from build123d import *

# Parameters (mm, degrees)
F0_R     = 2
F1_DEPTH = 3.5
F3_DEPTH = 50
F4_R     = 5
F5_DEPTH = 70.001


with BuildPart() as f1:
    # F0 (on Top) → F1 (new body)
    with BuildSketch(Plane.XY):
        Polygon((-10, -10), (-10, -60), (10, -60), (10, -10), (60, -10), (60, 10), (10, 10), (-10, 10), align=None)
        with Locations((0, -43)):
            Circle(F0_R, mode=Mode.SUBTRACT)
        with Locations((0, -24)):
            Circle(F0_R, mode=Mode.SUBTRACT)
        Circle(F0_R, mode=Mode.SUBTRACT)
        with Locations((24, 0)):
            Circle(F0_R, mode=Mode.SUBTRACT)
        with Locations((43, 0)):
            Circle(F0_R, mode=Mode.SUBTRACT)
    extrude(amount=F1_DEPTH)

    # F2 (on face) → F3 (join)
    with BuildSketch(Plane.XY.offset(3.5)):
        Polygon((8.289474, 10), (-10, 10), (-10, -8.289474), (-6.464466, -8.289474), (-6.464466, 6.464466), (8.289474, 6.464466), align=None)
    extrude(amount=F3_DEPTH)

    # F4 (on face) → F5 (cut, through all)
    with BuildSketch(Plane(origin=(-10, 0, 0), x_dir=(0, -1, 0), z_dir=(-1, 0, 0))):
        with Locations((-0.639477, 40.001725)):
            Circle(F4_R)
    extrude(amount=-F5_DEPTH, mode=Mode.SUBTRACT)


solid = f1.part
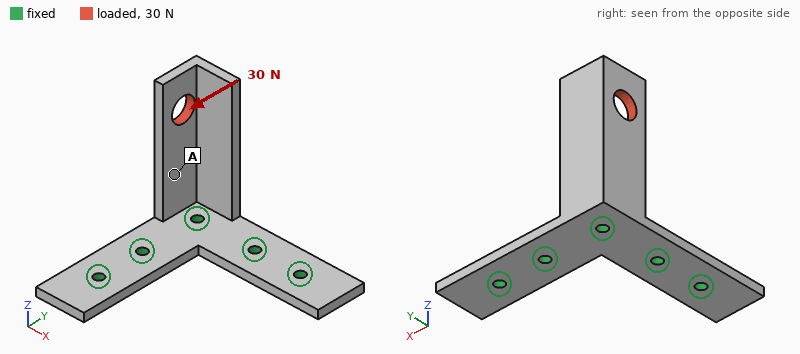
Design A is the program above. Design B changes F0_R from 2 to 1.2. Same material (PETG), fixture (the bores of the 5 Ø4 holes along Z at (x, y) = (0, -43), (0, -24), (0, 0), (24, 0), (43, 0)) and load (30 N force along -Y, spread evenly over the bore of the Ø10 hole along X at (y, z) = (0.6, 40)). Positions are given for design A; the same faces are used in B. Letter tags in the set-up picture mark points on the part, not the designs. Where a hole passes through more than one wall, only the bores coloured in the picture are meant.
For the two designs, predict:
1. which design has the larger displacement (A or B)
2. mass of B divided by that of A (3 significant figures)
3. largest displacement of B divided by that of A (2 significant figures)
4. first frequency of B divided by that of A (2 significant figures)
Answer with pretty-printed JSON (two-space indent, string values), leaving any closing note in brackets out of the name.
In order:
{
  "which design has the larger displacement": "B",
  "mass of B divided by that of A": "1.01",
  "largest displacement of B divided by that of A": "1.2",
  "first frequency of B divided by that of A": "0.92"
}
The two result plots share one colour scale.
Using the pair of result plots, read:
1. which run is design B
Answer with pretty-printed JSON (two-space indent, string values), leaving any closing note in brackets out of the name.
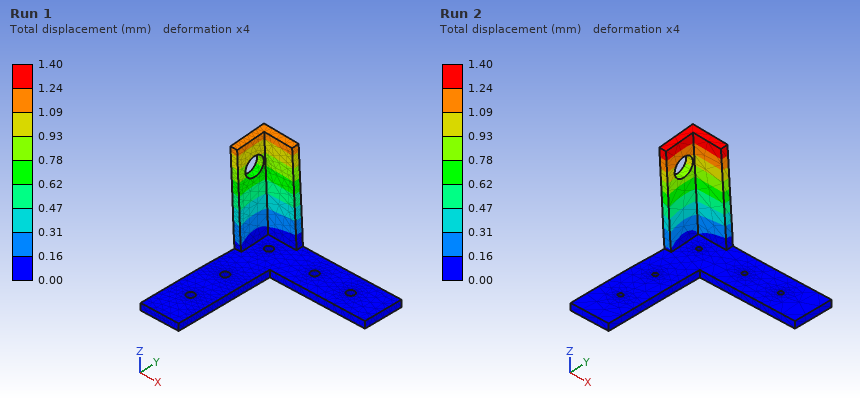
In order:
{
  "which run is design B": "Run 2"
}
